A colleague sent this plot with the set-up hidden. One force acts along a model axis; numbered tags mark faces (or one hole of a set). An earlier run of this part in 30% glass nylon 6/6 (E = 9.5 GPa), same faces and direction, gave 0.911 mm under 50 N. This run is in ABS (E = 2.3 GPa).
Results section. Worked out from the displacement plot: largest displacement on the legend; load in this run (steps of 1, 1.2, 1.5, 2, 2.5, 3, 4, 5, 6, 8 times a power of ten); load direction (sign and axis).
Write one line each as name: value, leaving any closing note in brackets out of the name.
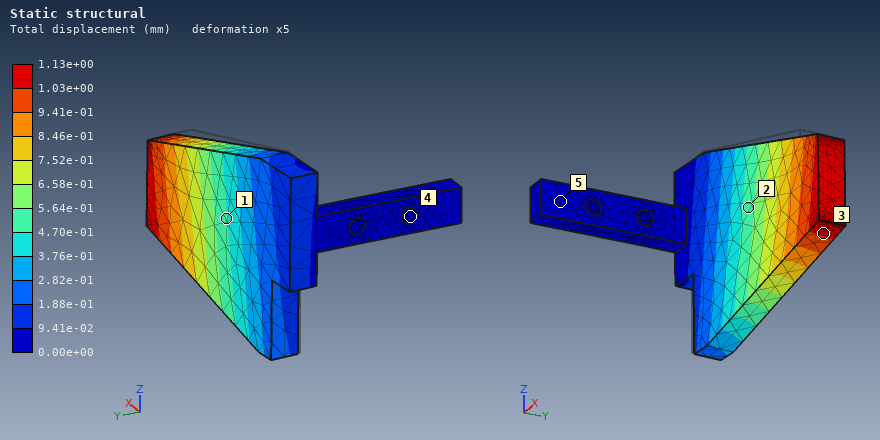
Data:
largest displacement on the legend: 1.13e+00 mm
load in this run: 15 N
load direction: +Y
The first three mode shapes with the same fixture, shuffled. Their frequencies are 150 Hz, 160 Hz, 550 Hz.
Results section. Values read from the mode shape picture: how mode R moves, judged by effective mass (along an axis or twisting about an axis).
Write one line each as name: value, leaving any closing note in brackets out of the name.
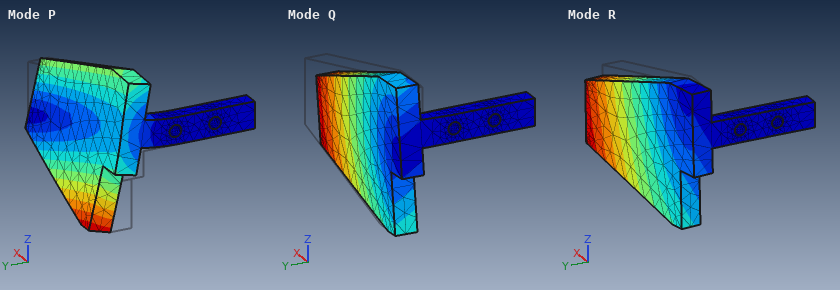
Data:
how mode R moves, judged by effective mass: along Y
